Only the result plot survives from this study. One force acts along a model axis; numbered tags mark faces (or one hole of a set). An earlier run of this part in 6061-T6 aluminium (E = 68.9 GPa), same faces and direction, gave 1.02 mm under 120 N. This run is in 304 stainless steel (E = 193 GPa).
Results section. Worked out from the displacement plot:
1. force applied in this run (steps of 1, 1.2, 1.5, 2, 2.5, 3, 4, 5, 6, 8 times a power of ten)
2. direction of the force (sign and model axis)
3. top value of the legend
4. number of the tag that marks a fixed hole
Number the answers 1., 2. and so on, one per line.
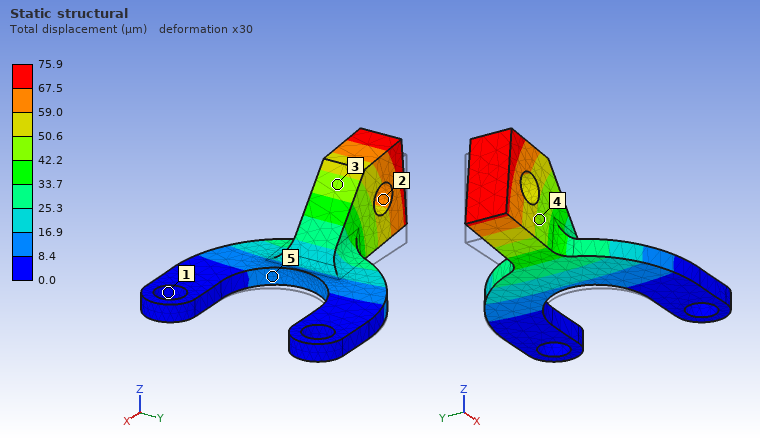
1. 25 N
2. +Z
3. 75.9 µm
4. 1
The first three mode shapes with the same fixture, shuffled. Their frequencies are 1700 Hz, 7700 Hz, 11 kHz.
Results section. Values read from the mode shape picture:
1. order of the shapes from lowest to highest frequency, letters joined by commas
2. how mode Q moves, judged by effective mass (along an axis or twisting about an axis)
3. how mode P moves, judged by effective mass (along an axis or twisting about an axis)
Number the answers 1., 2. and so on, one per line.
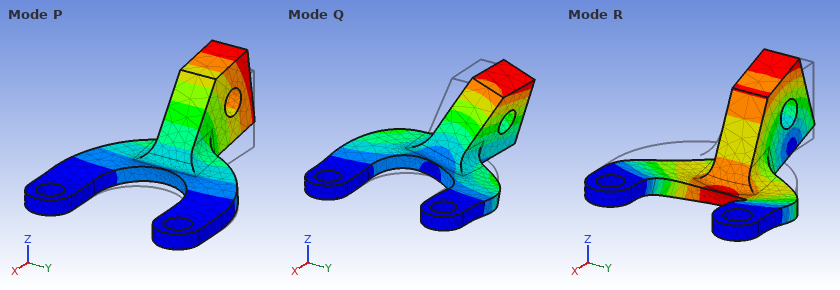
1. P, Q, R
2. along Y
3. along Z
